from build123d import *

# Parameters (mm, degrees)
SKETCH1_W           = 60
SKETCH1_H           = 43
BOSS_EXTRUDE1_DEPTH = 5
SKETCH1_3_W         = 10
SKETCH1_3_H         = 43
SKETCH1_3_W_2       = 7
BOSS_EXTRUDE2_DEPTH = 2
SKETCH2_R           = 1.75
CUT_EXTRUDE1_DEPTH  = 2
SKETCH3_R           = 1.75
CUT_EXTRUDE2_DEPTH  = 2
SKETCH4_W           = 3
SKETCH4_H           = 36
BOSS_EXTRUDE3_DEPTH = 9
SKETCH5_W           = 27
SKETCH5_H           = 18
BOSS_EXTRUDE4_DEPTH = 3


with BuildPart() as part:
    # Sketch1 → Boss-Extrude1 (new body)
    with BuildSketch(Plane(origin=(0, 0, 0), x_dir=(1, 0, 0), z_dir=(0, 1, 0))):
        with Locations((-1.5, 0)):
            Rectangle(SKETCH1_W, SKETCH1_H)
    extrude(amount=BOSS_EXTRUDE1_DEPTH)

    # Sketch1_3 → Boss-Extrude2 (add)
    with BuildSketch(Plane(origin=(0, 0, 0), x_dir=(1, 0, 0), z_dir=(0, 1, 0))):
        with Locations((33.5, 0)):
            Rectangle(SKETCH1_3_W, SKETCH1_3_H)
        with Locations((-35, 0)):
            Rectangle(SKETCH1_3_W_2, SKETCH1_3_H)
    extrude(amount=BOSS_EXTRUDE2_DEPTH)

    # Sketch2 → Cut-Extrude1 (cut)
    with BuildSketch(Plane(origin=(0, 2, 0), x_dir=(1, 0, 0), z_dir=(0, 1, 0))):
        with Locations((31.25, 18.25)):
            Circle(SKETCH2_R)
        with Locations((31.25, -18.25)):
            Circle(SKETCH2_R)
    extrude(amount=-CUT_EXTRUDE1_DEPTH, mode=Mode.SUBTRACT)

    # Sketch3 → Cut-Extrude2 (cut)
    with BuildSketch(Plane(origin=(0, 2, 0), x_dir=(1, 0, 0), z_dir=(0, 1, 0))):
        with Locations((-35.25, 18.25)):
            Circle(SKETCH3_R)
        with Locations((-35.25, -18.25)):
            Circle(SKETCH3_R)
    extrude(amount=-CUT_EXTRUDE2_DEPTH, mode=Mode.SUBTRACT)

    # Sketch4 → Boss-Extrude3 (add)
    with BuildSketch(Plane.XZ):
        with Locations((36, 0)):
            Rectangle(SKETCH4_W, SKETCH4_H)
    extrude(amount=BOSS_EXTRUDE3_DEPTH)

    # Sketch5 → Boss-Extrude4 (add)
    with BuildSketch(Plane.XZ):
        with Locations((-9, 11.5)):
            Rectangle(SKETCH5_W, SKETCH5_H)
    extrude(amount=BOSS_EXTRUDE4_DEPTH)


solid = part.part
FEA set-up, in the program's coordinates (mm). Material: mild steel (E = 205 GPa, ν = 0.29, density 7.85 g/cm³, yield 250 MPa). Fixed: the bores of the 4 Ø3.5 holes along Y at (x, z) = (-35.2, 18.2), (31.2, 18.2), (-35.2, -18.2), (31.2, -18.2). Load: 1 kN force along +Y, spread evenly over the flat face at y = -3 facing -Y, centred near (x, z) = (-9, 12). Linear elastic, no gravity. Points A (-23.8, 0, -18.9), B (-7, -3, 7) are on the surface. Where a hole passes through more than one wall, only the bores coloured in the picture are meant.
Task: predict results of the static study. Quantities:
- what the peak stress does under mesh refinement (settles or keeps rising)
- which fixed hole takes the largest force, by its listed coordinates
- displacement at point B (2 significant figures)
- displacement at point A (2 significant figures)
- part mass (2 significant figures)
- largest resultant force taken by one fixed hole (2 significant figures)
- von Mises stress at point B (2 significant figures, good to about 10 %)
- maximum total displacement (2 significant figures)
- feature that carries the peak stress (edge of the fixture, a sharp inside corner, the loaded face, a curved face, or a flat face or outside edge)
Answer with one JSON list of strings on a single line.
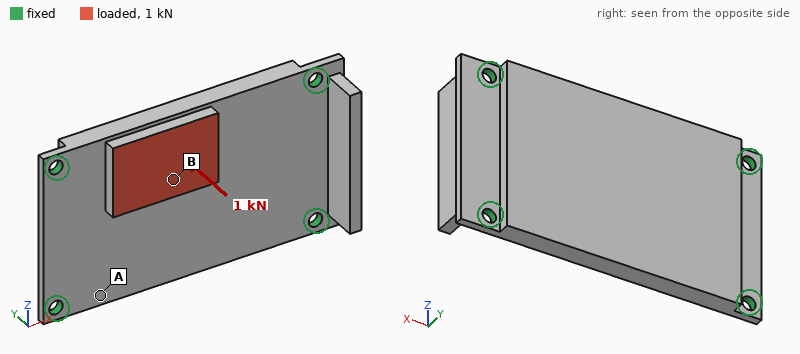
["keeps rising", "(-35.2, 18.2)", "25 µm", "5.7 µm", "130 g", "700 N", "32 MPa", "33 µm", "edge of the fixture"]
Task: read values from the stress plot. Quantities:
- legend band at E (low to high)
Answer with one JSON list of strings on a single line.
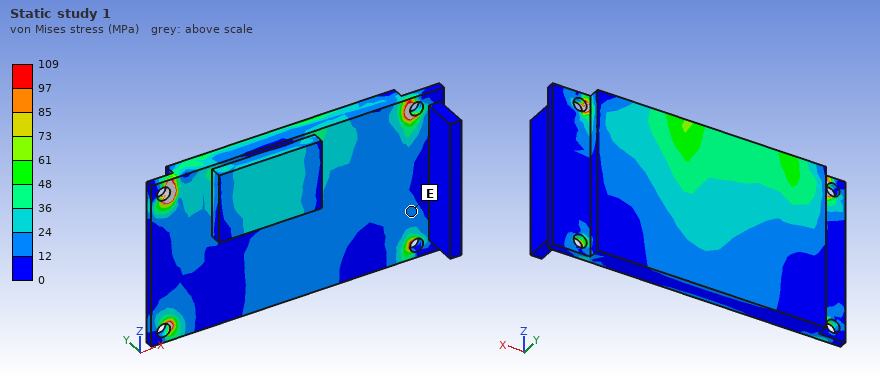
["12 to 24 MPa"]
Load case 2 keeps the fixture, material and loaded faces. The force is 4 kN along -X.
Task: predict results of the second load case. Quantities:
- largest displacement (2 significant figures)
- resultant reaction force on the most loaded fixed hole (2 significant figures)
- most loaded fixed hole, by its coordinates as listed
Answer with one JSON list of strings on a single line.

["22 µm", "1.6 kN", "(-35.2, 18.2)"]
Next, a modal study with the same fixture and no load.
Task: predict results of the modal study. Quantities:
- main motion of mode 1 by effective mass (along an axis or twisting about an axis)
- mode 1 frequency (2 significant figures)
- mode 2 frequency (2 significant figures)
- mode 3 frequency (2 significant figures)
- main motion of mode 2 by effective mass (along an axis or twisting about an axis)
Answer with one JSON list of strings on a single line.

["along Y", "3800 Hz", "6400 Hz", "9000 Hz", "twisting about X"]
